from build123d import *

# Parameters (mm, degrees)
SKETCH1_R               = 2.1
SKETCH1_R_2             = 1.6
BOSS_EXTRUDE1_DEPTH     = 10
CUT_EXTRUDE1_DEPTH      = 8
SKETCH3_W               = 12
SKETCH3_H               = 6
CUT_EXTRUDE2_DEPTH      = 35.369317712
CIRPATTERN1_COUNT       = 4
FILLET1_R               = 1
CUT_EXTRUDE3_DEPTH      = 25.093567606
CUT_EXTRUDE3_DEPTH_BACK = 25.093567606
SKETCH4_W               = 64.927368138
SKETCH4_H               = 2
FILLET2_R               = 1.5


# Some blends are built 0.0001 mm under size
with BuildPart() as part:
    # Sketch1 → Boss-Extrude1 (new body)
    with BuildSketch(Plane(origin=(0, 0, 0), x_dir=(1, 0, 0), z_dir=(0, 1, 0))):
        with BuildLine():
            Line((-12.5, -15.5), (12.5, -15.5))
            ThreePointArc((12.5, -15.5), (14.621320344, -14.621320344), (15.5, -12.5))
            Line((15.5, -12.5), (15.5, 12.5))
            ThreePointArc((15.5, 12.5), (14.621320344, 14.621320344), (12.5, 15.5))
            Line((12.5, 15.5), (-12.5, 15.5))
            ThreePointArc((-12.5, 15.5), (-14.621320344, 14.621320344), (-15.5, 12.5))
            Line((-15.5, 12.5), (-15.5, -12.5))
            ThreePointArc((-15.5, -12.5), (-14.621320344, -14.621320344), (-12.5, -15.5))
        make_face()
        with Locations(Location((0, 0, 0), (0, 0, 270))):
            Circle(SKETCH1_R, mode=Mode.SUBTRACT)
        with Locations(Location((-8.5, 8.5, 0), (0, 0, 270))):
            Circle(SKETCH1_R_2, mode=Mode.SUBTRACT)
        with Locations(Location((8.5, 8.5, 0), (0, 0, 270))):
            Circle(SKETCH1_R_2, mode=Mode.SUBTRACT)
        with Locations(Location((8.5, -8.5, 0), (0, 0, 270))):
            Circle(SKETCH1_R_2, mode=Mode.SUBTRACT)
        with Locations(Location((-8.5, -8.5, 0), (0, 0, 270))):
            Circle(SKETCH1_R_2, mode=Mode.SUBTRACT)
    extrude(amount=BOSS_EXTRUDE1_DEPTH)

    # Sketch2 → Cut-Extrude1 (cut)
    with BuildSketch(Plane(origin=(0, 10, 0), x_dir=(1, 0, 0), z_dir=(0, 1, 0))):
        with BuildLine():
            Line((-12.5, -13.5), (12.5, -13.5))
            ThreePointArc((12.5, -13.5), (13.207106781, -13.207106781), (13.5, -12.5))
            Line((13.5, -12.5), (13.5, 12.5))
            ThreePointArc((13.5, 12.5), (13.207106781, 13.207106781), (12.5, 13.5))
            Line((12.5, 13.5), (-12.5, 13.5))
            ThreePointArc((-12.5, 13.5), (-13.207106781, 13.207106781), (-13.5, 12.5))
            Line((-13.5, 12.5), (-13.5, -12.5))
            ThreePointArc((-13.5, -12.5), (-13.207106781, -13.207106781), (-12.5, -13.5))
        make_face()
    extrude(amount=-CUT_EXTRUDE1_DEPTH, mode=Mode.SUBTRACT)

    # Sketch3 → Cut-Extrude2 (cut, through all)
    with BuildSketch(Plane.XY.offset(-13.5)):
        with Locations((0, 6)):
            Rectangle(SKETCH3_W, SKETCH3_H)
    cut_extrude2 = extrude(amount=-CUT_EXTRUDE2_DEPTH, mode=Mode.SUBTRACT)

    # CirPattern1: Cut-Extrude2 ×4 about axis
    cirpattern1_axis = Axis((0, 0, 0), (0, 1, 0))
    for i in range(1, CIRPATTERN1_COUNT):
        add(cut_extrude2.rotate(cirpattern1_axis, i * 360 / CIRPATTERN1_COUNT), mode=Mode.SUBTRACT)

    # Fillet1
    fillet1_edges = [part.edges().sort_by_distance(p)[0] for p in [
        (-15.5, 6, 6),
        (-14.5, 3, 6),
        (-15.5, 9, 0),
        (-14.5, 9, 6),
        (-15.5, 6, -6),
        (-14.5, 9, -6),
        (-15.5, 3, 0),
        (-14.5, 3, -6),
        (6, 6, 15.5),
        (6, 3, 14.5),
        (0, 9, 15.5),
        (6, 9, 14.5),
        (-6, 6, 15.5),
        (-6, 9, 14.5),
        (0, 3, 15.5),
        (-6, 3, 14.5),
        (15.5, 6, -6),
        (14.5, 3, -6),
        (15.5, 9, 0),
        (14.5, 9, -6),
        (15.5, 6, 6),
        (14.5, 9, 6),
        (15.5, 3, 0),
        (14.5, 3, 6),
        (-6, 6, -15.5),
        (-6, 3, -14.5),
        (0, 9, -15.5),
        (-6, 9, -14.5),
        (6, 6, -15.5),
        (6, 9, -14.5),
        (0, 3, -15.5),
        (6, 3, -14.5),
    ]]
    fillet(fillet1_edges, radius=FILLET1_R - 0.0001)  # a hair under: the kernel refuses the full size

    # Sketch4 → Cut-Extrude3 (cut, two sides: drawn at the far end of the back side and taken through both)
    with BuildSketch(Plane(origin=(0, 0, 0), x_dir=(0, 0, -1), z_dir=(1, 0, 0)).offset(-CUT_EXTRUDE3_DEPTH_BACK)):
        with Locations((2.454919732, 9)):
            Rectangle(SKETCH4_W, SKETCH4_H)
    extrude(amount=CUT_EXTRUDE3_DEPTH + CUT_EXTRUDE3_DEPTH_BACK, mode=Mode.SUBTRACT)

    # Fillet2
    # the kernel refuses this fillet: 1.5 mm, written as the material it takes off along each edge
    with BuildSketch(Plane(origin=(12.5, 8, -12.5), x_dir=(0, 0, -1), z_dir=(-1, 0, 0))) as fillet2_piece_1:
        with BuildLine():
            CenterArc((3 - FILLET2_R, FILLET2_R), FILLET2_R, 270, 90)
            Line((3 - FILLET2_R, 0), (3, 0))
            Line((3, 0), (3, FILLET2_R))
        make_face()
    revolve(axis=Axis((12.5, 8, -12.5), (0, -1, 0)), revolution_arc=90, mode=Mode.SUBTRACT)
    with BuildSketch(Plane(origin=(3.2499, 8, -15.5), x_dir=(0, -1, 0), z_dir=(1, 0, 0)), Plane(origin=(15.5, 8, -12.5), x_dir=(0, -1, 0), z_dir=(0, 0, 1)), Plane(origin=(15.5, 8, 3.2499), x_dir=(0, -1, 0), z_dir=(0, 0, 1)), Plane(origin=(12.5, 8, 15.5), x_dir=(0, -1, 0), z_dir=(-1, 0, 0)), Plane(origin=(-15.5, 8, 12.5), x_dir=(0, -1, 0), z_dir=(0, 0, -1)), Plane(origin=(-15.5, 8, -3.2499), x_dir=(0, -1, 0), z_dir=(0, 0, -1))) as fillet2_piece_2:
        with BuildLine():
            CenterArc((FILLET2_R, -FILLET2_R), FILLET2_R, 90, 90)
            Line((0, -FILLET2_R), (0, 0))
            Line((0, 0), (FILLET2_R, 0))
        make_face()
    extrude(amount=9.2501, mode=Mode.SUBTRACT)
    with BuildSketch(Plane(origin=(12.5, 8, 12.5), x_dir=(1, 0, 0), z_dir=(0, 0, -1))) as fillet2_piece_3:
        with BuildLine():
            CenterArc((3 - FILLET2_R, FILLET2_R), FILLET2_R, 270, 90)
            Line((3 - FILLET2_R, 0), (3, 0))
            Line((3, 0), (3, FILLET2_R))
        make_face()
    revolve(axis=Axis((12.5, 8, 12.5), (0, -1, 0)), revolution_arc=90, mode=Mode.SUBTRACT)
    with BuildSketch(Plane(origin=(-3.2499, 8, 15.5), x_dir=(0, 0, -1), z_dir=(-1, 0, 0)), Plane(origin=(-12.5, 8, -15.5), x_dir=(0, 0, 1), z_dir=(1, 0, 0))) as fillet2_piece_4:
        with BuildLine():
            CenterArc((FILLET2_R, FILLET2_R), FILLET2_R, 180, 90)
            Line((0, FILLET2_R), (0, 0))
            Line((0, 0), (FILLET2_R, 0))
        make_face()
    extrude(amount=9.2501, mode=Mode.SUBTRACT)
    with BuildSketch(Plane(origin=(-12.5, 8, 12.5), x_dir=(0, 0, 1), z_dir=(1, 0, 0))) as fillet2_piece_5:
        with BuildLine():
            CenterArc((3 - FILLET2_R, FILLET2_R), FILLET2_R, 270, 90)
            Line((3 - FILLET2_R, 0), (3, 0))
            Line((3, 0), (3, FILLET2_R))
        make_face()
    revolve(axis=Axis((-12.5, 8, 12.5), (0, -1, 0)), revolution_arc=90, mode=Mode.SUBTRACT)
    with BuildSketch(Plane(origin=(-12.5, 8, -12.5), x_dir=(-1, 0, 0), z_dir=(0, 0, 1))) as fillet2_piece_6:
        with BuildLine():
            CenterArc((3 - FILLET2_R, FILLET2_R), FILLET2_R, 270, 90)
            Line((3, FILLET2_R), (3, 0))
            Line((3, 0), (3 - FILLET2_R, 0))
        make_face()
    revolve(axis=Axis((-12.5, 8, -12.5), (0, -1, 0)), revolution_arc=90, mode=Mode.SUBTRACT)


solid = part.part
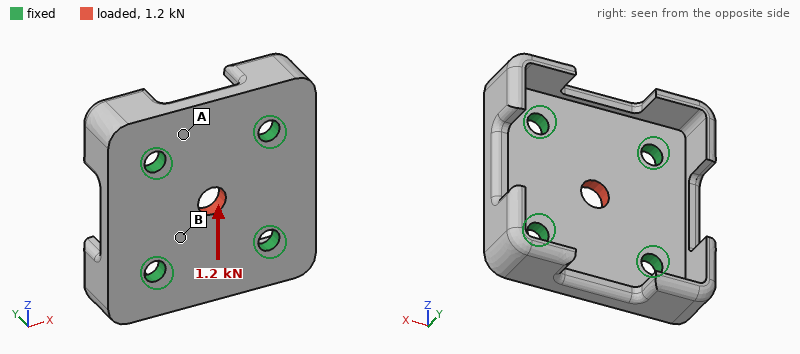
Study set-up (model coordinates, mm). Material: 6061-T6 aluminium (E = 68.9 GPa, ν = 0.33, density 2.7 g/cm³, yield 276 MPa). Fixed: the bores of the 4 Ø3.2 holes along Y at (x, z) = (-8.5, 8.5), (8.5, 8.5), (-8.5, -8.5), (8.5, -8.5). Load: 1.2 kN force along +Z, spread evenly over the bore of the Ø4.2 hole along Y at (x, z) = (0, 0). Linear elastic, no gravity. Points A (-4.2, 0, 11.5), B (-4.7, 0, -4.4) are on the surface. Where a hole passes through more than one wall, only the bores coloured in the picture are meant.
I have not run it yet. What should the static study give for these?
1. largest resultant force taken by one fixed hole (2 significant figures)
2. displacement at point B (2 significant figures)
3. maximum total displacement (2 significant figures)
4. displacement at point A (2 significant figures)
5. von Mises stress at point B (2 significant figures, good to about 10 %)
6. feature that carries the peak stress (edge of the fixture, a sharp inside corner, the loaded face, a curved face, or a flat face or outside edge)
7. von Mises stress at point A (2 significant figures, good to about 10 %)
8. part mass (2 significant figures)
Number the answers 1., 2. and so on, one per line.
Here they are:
1. 320 N
2. 1.8 µm
3. 4.8 µm
4. 1.4 µm
5. 26 MPa
6. the loaded face
7. 12 MPa
8. 7.1 g
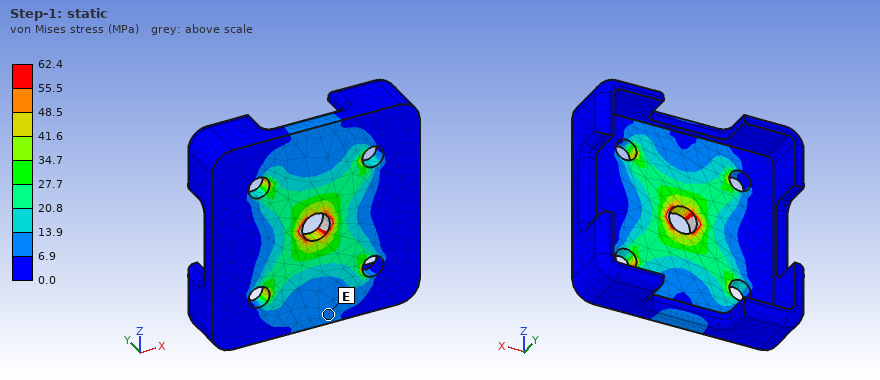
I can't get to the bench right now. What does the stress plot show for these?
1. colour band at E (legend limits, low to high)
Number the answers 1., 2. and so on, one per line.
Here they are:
1. 6.9 to 13.9 MPa
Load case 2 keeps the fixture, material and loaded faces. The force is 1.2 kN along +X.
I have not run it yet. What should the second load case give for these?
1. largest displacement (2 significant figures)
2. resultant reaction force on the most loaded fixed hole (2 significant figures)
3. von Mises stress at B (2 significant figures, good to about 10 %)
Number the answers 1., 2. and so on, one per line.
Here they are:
1. 4.8 µm
2. 320 N
3. 26 MPa
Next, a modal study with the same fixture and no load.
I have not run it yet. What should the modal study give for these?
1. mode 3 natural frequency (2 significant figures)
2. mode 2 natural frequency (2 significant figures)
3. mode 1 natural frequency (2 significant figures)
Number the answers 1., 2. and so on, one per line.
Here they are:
1. 18 kHz
2. 18 kHz
3. 18 kHz
